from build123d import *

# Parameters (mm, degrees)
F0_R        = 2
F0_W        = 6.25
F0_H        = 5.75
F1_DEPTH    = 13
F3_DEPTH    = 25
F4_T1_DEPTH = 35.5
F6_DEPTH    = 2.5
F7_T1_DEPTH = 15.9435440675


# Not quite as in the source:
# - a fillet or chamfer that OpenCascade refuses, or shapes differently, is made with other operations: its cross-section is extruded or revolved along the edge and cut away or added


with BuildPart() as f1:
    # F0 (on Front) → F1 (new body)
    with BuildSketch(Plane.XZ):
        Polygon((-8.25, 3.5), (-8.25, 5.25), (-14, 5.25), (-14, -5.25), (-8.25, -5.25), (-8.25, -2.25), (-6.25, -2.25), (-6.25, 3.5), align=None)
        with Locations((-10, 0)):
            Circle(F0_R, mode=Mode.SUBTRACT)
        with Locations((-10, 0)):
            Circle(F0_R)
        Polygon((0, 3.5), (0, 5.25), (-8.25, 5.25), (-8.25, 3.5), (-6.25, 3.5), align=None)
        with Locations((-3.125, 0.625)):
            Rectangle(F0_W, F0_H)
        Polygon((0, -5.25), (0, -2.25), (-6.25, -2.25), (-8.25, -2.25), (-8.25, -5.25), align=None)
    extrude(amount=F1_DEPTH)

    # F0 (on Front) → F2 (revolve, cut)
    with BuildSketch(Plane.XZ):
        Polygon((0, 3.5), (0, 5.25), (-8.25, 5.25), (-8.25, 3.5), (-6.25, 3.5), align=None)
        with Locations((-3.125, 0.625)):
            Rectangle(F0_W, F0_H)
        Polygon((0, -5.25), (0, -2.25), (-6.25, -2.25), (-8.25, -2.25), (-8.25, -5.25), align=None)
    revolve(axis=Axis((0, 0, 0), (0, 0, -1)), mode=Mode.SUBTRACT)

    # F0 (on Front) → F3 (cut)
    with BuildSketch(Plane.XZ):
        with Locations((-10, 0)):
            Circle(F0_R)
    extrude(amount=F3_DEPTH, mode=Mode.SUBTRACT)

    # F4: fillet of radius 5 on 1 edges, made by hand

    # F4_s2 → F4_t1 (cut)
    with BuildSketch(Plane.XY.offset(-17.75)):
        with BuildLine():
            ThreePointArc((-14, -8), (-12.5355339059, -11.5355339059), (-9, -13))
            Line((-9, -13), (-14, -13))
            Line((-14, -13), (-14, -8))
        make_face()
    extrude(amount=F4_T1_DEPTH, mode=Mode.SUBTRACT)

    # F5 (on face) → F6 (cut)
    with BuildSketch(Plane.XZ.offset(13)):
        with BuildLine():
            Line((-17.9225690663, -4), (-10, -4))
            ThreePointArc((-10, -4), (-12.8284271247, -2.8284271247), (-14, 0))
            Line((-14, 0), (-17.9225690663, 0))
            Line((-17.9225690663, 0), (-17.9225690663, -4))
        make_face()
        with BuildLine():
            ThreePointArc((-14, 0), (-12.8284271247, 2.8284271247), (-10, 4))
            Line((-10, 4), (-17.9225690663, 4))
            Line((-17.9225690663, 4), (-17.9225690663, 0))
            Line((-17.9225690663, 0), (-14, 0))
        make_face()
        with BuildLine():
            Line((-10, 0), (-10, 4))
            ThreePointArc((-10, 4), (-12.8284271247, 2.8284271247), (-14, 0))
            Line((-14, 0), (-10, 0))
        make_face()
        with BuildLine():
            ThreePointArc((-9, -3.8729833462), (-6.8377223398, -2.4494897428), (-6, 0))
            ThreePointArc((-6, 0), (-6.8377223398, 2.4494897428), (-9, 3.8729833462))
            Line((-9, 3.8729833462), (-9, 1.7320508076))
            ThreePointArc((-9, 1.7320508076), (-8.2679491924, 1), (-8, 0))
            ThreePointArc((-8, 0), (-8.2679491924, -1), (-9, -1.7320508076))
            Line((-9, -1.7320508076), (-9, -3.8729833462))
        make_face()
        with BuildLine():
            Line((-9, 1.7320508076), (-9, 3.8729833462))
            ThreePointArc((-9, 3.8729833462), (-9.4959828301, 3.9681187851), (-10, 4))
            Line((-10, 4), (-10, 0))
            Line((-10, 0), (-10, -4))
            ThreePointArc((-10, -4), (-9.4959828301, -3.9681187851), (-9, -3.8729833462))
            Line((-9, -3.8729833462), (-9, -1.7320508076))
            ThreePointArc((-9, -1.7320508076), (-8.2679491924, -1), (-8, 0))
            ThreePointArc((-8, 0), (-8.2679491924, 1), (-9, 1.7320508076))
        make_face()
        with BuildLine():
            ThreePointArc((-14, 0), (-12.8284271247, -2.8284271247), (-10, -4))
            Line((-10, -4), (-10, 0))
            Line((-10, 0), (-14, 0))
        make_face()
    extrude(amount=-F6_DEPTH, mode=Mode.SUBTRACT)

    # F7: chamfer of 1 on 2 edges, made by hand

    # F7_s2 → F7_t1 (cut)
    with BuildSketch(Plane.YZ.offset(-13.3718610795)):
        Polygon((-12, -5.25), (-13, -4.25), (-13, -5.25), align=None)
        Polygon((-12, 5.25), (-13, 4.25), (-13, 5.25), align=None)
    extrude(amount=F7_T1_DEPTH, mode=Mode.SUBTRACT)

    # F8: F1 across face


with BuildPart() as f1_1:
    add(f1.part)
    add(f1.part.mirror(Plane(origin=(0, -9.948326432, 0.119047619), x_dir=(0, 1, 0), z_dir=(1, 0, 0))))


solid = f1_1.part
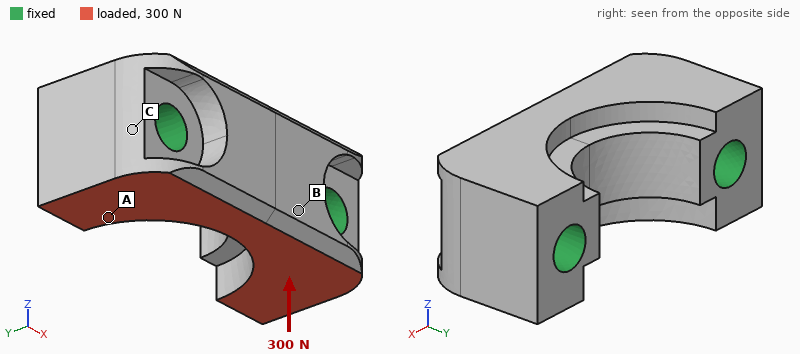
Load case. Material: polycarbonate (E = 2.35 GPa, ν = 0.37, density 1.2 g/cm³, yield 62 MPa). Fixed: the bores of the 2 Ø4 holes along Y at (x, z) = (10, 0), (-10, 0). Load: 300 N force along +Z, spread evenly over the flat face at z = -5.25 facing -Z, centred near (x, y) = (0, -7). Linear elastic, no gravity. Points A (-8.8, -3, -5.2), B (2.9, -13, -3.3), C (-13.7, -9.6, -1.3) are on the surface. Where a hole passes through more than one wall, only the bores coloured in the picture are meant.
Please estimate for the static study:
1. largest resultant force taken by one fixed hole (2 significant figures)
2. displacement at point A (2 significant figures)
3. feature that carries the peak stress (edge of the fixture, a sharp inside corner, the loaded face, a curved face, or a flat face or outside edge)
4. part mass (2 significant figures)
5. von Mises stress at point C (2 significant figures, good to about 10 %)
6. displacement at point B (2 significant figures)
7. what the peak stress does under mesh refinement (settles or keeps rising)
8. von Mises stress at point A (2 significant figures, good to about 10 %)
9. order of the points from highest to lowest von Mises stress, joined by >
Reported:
150 N
2.4 µm
edge of the fixture
2.8 g
1.1 MPa
13 µm
keeps rising
1.8 MPa
A > C > B
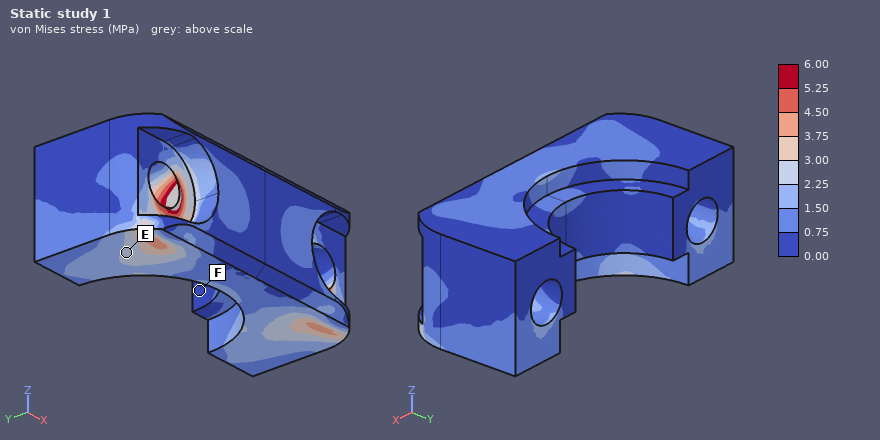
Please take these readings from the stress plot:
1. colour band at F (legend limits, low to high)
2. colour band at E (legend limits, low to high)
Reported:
0.00 to 0.75 MPa
2.25 to 3.00 MPa
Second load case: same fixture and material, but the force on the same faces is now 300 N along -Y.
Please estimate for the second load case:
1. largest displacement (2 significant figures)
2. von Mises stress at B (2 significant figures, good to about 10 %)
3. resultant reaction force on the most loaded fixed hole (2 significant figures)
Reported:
29 µm
2.2 MPa
150 N
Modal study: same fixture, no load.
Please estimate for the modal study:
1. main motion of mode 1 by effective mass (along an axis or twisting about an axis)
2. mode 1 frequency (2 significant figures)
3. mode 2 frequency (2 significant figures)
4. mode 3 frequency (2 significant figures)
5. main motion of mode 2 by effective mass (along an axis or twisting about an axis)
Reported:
along Z
15 kHz
20 kHz
24 kHz
along Y
